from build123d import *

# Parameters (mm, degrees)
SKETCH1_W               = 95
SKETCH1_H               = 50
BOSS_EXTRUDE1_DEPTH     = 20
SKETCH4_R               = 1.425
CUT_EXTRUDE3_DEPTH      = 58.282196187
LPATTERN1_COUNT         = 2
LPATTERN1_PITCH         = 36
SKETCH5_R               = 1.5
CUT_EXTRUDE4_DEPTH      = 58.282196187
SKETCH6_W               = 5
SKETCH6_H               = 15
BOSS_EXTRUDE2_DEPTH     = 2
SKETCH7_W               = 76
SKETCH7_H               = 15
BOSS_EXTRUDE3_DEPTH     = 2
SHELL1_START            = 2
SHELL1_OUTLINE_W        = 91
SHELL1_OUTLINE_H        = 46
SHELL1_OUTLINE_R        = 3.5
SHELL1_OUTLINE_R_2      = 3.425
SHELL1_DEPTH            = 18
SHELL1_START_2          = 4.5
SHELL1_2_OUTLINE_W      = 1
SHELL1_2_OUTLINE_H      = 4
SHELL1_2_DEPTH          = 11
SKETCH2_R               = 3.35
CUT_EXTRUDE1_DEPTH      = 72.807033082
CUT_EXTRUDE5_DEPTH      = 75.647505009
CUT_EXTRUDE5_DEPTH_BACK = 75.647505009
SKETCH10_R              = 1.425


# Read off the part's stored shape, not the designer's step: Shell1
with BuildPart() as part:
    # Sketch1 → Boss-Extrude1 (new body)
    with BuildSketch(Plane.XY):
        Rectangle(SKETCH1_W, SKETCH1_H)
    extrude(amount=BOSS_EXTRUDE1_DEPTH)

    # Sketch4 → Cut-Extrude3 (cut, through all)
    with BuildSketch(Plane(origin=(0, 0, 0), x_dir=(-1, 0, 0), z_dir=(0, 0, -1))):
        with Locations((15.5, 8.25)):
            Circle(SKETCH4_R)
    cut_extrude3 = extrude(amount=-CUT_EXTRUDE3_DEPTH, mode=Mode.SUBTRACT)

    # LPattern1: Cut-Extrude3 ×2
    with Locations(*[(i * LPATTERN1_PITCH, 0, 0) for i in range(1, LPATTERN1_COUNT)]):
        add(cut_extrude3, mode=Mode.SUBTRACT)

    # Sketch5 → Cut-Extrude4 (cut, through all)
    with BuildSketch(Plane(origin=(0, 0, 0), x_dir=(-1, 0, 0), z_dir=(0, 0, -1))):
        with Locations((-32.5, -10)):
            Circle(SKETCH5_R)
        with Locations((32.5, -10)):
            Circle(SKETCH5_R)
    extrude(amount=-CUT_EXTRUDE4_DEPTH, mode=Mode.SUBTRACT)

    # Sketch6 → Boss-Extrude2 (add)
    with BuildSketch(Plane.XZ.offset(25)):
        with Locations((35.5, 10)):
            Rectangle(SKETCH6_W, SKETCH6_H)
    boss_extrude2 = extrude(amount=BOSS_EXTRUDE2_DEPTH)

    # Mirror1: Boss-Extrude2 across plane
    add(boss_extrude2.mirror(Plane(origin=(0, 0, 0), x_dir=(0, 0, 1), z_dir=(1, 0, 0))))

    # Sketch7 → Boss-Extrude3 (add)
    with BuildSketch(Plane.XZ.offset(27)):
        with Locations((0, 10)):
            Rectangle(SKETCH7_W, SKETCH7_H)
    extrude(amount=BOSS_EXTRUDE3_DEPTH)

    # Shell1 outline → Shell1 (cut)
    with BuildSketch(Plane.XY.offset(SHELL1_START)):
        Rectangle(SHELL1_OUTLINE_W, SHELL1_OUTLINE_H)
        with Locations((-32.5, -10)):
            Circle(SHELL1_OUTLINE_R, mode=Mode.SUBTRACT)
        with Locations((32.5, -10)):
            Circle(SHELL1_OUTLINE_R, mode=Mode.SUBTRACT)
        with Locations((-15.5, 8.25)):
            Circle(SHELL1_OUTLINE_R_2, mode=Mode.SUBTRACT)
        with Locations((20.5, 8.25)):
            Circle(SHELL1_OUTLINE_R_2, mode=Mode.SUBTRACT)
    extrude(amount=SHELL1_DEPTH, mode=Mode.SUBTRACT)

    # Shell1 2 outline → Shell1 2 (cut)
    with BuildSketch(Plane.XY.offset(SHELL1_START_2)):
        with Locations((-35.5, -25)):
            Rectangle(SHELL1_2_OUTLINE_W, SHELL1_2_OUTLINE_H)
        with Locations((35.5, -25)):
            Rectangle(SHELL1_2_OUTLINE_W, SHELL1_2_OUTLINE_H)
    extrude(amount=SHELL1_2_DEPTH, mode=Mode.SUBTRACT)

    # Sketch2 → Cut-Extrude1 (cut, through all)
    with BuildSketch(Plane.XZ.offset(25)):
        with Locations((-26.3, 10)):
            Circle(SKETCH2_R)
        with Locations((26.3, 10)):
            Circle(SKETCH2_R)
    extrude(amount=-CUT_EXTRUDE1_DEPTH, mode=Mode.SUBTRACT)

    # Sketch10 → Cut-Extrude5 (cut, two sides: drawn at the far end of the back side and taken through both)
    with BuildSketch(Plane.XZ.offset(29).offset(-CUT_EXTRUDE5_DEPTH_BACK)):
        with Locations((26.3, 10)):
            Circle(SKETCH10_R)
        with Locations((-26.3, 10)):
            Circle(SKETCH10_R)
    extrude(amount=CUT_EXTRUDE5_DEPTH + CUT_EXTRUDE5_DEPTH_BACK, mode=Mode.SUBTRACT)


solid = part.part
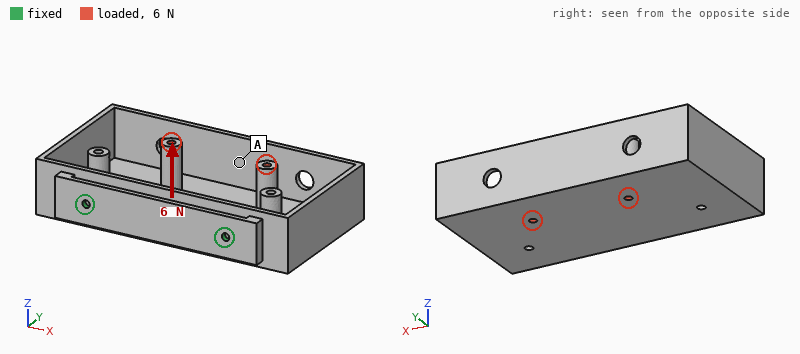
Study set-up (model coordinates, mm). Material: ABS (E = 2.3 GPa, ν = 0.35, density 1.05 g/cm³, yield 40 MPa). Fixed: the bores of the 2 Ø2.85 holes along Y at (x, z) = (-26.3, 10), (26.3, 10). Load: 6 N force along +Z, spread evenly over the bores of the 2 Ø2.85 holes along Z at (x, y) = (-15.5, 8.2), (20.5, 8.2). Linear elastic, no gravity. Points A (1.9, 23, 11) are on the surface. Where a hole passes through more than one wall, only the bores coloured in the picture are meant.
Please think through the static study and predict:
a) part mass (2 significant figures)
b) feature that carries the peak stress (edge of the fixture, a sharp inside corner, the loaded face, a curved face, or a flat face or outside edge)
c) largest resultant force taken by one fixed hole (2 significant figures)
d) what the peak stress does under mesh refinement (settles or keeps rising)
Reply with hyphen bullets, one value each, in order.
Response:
- 25 g
- edge of the fixture
- 5.5 N
- keeps rising
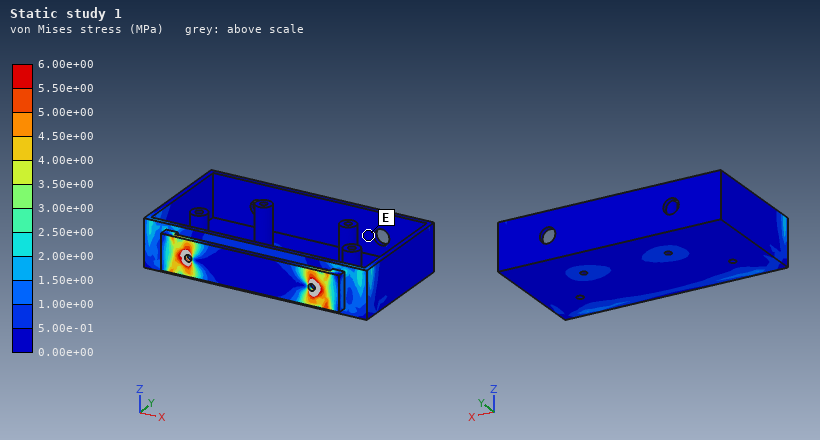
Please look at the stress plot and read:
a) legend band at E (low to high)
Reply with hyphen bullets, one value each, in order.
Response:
- 0.00e+00 to 5.00e-01 MPa
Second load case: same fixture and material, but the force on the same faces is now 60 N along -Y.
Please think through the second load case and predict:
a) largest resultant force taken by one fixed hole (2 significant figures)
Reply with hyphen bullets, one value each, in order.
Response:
- 49 N
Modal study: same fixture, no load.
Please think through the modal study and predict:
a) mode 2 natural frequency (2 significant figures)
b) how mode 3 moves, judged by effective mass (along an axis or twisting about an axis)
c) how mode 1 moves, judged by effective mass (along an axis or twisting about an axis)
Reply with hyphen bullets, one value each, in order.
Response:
- 210 Hz
- along X
- along Z
